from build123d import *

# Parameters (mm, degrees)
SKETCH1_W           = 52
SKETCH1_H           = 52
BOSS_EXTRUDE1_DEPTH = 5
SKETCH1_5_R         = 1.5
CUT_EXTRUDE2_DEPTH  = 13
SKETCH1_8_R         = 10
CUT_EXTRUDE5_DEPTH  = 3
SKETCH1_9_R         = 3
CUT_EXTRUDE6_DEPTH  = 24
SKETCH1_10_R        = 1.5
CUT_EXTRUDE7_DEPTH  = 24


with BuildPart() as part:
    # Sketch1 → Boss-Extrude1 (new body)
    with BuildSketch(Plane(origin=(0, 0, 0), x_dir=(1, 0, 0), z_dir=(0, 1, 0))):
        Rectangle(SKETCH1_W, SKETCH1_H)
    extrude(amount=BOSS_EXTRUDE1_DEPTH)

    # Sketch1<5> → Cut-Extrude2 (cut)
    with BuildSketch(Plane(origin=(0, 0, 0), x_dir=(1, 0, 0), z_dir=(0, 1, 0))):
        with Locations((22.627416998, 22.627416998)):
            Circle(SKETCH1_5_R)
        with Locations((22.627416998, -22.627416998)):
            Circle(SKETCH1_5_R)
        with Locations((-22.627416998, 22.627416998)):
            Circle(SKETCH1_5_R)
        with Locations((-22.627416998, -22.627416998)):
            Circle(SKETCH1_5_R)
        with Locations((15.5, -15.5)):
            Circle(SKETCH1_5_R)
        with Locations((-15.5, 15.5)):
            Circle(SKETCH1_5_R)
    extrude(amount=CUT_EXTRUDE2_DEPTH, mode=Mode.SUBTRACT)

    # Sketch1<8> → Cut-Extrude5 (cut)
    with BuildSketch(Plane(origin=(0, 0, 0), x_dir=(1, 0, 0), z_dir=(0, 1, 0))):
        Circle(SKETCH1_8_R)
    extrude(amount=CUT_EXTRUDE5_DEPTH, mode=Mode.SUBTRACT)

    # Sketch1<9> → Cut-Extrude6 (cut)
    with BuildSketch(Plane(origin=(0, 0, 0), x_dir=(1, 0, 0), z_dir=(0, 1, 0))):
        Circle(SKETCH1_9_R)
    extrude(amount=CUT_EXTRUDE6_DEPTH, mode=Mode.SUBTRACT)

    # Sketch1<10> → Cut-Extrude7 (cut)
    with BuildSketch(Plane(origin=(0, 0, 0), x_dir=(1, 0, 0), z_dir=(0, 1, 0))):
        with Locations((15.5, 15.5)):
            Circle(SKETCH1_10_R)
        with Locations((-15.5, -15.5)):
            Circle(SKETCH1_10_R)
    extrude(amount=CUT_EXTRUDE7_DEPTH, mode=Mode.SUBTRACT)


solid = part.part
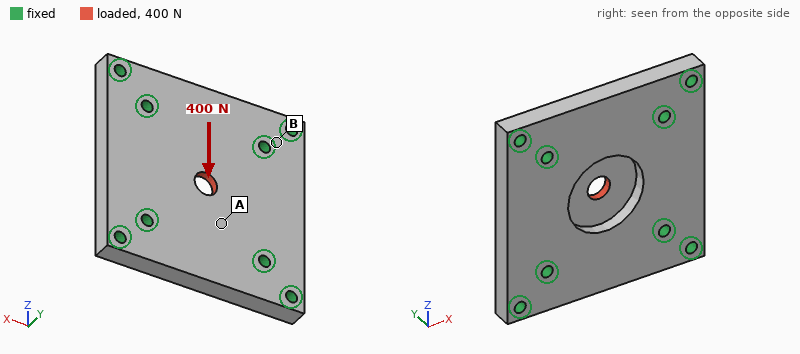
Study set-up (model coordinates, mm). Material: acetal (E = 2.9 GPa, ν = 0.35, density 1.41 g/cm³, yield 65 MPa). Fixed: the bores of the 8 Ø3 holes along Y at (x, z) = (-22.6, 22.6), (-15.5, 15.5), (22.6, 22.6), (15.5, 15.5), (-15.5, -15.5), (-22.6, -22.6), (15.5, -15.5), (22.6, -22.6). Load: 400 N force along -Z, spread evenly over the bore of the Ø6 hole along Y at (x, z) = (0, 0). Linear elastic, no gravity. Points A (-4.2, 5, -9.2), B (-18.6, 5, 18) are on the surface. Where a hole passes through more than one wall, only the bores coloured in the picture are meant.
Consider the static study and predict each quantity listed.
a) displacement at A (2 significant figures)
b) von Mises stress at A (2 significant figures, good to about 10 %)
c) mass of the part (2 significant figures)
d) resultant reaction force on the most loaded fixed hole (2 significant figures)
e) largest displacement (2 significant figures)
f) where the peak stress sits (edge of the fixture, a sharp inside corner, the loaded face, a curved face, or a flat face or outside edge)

19 µm
4.3 MPa
17 g
93 N
37 µm
the loaded face
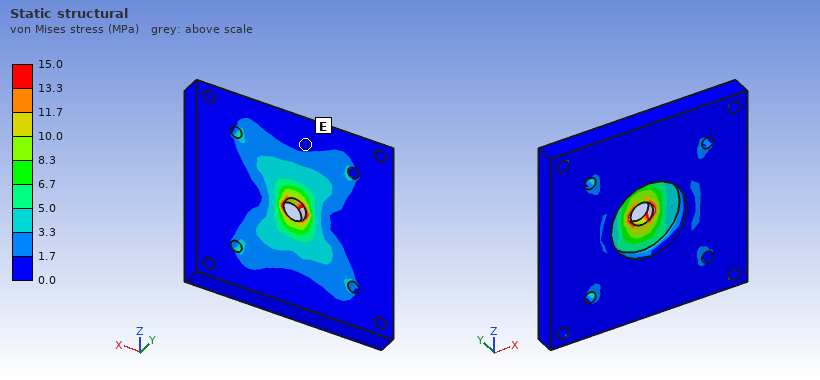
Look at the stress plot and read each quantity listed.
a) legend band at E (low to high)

0.0 to 1.7 MPa
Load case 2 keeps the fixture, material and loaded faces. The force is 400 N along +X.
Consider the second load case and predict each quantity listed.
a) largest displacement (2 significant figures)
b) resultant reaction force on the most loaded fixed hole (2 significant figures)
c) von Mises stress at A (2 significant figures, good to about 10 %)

37 µm
93 N
2.6 MPa
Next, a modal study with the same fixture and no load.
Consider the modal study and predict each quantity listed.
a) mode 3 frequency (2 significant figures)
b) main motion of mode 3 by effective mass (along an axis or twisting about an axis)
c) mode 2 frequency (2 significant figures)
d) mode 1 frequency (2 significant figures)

5900 Hz
twisting about X
5500 Hz
5400 Hz
